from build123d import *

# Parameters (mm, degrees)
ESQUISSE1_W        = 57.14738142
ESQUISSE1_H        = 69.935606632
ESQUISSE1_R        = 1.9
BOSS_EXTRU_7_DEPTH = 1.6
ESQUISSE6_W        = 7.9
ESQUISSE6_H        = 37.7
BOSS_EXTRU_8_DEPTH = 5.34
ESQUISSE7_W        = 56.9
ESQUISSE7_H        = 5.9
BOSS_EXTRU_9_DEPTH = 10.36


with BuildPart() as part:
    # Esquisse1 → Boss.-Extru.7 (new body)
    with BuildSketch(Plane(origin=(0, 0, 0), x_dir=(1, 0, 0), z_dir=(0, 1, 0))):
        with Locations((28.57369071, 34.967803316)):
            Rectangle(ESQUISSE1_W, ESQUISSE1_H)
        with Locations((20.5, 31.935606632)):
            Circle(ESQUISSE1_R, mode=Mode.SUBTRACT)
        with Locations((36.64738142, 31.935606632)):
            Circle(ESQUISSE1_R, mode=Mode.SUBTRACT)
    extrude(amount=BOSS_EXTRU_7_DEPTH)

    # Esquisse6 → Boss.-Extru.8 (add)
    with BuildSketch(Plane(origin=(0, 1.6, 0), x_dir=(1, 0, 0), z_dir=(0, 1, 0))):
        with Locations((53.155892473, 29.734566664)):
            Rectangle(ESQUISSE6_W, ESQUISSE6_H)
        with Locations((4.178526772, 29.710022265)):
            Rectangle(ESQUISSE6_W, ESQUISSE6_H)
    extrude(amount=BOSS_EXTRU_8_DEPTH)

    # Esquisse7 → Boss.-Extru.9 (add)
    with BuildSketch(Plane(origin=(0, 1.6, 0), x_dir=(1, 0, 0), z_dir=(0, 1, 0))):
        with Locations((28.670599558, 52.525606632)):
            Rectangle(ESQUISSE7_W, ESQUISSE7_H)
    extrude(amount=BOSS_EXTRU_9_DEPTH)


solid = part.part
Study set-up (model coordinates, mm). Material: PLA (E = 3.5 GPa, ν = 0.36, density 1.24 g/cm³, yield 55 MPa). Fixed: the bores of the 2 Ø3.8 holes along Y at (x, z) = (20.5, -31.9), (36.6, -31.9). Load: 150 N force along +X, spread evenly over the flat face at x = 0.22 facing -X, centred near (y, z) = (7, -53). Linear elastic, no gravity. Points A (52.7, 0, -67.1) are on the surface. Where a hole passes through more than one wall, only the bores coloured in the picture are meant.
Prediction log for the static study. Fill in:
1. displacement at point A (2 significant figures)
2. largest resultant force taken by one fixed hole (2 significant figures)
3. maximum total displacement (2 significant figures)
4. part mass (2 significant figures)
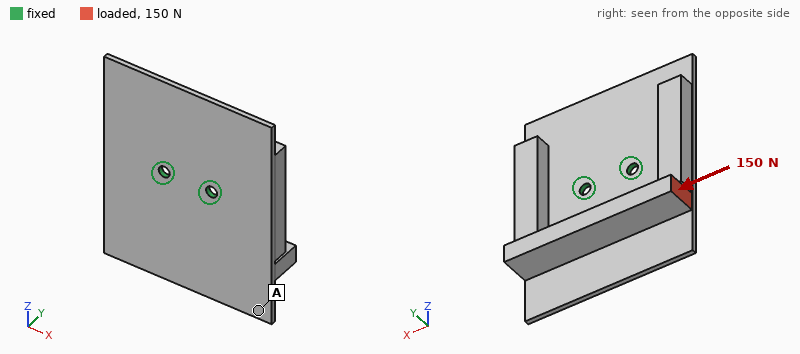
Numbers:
0.82 mm
180 N
1.0 mm
16 g
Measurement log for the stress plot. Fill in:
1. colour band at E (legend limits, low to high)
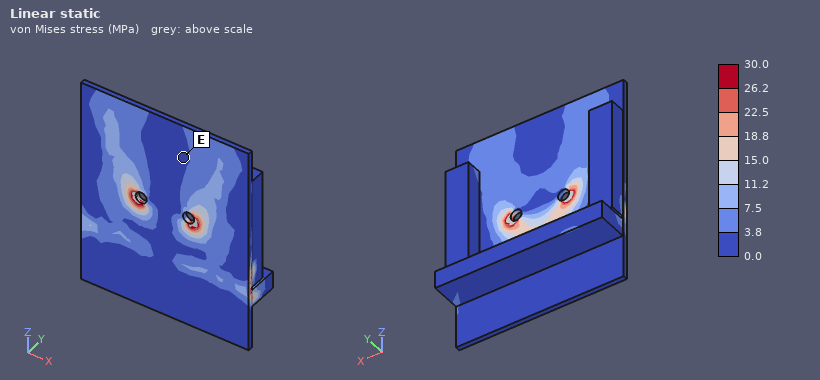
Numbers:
0.0 to 3.8 MPa
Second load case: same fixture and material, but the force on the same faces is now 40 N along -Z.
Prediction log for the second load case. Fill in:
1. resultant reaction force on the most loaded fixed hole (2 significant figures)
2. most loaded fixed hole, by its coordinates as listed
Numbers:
81 N
(20.5, -31.9)
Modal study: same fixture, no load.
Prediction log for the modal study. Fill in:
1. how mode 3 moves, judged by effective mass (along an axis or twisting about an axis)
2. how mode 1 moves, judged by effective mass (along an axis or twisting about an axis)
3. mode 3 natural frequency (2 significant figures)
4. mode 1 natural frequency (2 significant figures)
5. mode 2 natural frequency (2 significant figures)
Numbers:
along Y
along Y
680 Hz
270 Hz
460 Hz
